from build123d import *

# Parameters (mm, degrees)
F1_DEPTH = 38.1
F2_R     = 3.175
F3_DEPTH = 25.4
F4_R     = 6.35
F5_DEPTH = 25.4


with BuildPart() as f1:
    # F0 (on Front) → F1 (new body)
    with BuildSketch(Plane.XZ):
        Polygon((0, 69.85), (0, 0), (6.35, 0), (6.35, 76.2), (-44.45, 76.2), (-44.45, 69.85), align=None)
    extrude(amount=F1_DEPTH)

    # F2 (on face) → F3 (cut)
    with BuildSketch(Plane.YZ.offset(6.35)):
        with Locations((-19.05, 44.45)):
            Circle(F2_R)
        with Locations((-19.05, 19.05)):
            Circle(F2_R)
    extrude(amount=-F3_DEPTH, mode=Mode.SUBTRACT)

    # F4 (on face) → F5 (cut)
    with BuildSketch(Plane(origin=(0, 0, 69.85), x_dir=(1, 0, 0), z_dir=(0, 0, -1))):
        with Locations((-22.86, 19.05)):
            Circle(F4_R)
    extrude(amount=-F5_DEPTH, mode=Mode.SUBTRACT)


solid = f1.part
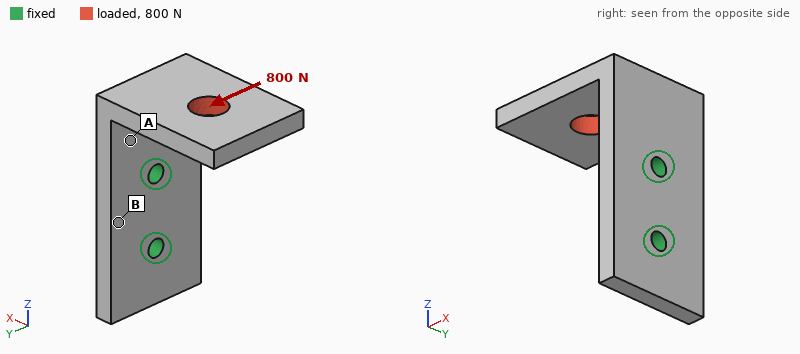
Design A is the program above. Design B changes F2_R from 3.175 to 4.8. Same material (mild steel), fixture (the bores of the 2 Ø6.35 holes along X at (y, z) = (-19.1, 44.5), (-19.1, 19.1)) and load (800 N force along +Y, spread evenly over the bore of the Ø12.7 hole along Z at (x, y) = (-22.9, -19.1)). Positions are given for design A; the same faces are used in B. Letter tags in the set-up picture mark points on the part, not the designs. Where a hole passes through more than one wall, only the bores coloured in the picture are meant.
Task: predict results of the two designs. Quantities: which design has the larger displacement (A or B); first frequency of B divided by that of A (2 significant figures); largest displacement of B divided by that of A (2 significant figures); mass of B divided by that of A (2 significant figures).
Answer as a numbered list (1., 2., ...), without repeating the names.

1. A
2. 1.0
3. 0.86
4. 0.98
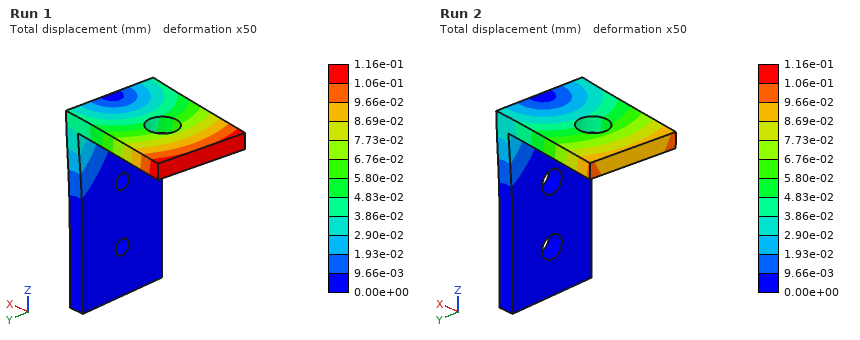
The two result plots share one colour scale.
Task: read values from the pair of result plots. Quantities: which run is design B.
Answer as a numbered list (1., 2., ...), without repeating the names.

1. Run 2
